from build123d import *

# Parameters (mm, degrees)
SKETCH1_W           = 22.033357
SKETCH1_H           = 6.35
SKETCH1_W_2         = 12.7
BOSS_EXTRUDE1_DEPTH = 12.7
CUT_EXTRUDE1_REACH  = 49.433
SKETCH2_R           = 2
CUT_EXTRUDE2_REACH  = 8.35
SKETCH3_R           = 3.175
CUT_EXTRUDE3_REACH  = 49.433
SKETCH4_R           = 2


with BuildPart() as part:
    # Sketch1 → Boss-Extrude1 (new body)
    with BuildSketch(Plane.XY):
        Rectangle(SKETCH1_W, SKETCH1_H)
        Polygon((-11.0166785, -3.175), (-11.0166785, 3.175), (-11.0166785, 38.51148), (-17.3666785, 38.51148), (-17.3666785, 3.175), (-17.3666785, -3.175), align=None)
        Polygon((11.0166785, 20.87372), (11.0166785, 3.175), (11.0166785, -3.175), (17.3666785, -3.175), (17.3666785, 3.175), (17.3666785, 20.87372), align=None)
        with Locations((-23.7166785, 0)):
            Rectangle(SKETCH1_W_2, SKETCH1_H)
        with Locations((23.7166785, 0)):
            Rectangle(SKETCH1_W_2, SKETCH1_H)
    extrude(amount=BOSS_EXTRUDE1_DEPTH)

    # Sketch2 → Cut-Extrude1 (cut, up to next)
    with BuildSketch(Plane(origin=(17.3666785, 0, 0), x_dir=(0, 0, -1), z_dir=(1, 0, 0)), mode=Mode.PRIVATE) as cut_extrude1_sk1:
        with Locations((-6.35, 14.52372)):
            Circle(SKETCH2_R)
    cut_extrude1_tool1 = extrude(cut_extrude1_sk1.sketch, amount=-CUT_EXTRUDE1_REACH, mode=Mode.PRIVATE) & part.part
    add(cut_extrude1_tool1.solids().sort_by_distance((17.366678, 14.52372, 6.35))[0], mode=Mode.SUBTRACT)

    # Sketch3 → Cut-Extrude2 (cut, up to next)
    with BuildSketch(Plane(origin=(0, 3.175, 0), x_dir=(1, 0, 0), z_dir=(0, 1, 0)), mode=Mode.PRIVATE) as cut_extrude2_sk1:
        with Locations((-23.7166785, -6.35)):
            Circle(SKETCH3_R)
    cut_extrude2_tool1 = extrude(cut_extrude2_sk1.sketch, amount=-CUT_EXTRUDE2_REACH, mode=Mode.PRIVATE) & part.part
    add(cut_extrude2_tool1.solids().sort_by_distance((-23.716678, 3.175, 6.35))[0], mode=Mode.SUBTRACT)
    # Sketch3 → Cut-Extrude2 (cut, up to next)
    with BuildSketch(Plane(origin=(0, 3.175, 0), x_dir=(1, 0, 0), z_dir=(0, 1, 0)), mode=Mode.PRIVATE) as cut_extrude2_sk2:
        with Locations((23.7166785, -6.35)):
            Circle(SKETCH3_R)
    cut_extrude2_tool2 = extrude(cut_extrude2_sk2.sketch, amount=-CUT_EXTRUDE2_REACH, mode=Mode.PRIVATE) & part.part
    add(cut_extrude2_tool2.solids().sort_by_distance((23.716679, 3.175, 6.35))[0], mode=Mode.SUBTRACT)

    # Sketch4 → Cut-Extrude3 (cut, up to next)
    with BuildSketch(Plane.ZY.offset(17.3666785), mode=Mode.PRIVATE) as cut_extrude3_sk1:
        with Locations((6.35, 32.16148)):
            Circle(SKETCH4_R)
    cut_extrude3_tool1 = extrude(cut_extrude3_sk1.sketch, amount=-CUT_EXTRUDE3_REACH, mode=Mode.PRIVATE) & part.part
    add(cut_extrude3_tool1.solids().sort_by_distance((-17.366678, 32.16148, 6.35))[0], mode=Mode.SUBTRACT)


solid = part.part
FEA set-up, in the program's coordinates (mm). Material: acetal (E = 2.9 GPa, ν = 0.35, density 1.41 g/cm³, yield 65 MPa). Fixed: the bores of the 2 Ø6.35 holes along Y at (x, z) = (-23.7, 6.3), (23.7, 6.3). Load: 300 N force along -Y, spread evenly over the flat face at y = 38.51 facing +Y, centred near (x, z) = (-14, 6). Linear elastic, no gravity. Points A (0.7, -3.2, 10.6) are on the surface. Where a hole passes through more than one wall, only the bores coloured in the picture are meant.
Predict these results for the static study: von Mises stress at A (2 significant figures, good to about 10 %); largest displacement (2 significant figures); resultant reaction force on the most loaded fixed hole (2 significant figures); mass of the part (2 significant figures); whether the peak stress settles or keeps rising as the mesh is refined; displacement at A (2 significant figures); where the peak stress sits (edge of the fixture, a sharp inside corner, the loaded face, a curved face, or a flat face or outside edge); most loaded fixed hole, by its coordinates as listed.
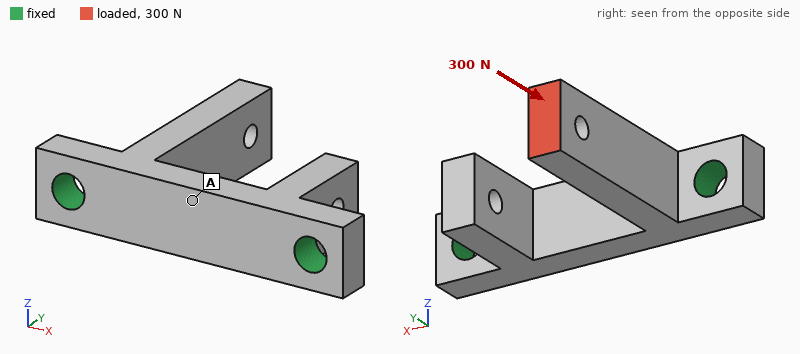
2.3 MPa
0.24 mm
270 N
12 g
keeps rising
0.061 mm
edge of the fixture
(-23.7, 6.3)
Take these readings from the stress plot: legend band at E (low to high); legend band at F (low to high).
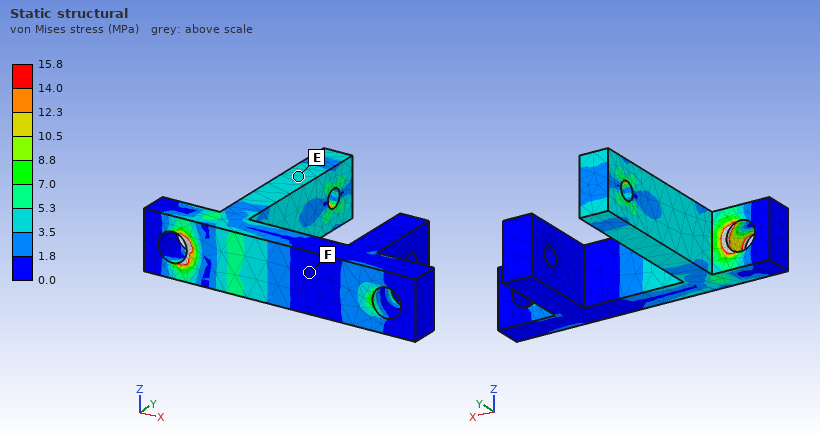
3.5 to 5.3 MPa
0.0 to 1.8 MPa
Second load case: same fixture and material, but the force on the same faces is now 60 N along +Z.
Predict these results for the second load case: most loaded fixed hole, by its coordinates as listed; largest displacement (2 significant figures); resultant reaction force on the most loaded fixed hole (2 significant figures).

(-23.7, 6.3)
0.82 mm
58 N
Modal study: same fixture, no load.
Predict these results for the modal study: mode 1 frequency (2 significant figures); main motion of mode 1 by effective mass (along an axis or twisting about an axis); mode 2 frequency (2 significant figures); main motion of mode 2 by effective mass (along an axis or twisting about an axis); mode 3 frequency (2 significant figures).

940 Hz
along X
1200 Hz
along Z
2700 Hz
